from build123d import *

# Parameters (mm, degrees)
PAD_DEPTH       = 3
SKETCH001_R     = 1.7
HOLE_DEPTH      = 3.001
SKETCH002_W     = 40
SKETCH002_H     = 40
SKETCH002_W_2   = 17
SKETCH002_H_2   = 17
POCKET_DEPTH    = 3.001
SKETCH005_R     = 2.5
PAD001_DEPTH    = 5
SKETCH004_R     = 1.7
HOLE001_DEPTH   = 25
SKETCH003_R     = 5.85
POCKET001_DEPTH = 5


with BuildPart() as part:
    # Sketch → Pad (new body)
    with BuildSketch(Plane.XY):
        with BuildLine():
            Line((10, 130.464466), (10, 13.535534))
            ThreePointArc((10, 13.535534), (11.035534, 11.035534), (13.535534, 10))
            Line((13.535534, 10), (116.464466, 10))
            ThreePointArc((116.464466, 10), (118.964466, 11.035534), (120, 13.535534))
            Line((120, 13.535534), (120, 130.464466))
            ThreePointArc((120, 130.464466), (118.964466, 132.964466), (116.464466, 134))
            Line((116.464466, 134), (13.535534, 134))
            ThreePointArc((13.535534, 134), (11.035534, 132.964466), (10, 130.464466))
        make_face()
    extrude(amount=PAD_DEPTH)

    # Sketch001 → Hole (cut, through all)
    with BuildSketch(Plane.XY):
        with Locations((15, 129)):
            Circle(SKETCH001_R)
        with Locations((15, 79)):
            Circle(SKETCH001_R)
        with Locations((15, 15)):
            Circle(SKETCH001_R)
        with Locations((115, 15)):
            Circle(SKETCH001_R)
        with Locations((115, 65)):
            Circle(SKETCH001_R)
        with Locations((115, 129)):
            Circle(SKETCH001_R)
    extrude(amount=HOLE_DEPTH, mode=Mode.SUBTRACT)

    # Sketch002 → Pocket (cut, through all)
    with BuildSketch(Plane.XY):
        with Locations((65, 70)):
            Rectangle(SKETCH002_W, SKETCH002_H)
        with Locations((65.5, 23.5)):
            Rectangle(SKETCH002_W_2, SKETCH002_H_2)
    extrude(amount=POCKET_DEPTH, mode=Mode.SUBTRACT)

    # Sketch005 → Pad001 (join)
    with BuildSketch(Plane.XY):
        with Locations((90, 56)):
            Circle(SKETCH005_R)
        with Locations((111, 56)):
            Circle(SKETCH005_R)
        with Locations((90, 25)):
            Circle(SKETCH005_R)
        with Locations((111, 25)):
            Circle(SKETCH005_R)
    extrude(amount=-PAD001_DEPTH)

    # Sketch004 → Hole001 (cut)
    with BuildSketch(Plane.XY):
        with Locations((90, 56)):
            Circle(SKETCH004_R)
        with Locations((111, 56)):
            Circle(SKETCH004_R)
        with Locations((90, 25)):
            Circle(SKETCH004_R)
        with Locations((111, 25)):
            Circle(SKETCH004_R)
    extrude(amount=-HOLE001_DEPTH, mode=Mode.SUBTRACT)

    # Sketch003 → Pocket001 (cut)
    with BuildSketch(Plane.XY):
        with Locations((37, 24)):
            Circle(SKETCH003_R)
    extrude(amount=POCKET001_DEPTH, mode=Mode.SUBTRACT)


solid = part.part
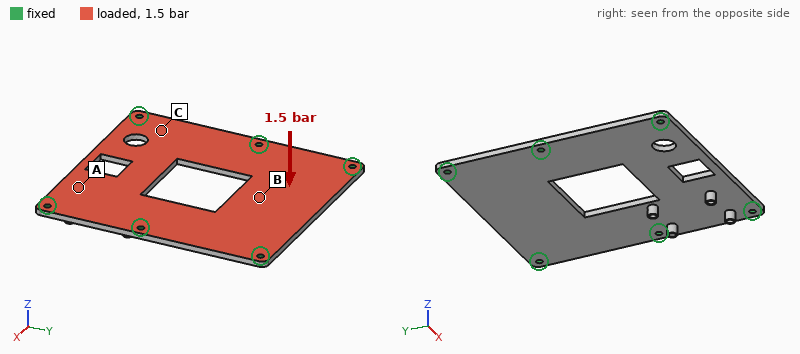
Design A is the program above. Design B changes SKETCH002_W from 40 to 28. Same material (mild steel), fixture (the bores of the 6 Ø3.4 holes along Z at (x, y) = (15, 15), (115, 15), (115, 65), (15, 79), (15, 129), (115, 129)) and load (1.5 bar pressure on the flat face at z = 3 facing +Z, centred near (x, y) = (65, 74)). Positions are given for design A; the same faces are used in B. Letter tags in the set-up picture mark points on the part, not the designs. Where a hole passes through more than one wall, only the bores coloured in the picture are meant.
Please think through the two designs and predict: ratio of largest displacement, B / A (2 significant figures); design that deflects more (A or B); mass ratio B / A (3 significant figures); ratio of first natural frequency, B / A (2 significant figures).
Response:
1.1
B
1.04
0.96
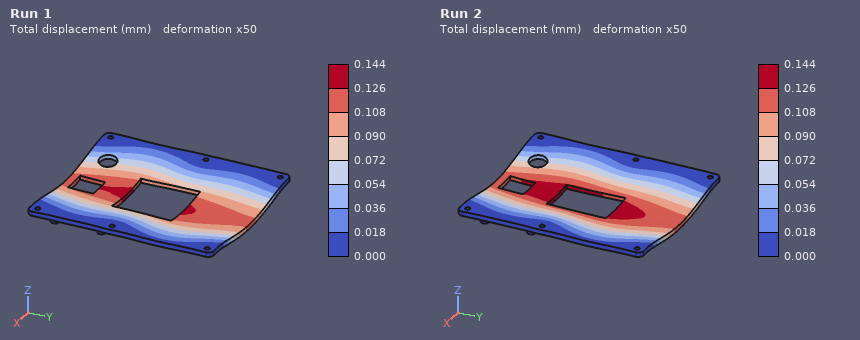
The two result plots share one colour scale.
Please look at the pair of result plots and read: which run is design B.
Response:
Run 2
